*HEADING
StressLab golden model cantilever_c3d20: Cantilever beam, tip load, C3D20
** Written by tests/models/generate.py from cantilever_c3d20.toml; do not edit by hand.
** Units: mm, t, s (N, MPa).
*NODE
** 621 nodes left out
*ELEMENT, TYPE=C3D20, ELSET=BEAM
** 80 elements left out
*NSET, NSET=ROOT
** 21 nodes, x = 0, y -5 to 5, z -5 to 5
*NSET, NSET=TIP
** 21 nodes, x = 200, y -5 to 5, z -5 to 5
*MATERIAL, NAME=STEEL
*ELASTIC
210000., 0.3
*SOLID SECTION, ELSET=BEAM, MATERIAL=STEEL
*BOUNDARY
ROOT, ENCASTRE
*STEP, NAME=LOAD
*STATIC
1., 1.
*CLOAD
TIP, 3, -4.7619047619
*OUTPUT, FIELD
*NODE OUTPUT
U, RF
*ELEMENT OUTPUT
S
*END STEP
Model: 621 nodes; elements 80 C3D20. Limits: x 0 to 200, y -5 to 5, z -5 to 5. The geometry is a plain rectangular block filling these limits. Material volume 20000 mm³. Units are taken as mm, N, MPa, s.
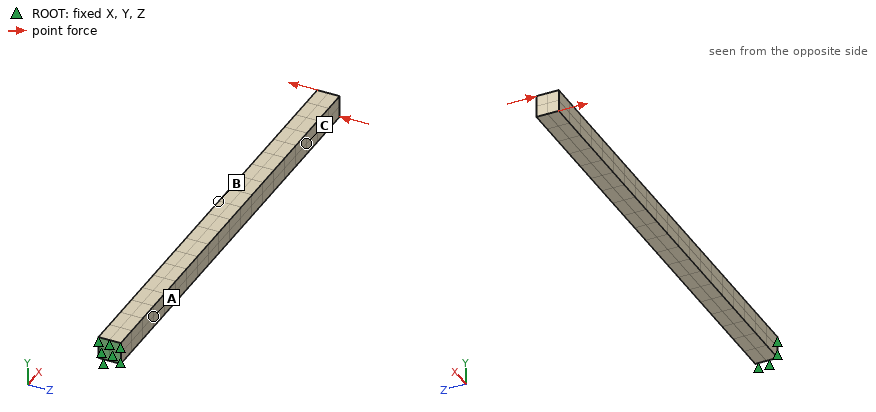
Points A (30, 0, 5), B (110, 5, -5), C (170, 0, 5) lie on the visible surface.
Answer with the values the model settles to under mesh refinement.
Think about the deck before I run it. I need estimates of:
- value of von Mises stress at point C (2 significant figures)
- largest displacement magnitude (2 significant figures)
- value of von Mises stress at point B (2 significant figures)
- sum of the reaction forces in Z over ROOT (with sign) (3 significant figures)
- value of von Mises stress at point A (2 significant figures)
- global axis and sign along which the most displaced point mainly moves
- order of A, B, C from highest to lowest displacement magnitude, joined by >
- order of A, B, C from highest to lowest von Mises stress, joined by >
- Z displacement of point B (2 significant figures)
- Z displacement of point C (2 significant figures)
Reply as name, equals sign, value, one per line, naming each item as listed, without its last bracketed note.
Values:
value of von Mises stress at point C = 18 MPa
largest displacement magnitude = 1.5 mm
value of von Mises stress at point B = 54 MPa
sum of the reaction forces in Z over ROOT (with sign) = 100 N
value of von Mises stress at point A = 100 MPa
global axis and sign along which the most displaced point mainly moves = -Z
order of A, B, C from highest to lowest displacement magnitude, joined by > = C > B > A
order of A, B, C from highest to lowest von Mises stress, joined by > = A > B > C
Z displacement of point B = -0.56 mm
Z displacement of point C = -1.2 mm
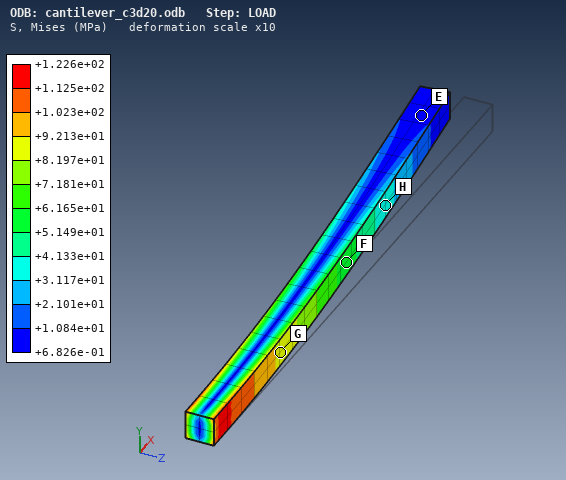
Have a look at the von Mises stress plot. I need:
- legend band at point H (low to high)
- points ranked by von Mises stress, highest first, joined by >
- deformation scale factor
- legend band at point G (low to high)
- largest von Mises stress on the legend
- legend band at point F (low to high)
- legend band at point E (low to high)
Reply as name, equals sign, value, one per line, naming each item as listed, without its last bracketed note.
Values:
legend band at point H = +3.117e+01 to +4.133e+01 MPa
points ranked by von Mises stress, highest first, joined by > = G > F > H > E
deformation scale factor = 10
legend band at point G = +8.197e+01 to +9.213e+01 MPa
largest von Mises stress on the legend = +1.226e+02 MPa
legend band at point F = +5.149e+01 to +6.165e+01 MPa
legend band at point E = +6.826e-01 to +1.084e+01 MPa
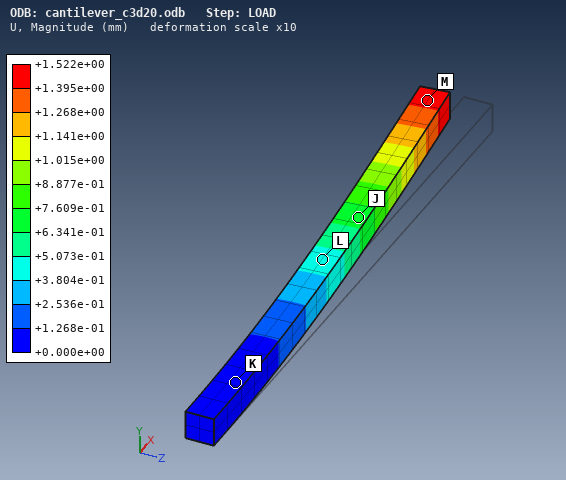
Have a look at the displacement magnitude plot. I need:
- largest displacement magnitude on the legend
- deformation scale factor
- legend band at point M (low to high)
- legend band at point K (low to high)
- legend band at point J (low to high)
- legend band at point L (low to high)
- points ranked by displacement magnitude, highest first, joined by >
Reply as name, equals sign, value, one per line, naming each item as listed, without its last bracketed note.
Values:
largest displacement magnitude on the legend = +1.522e+00 mm
deformation scale factor = 10
legend band at point M = +1.395e+00 to +1.522e+00 mm
legend band at point K = +0.000e+00 to +1.268e-01 mm
legend band at point J = +6.341e-01 to +7.609e-01 mm
legend band at point L = +3.804e-01 to +5.073e-01 mm
points ranked by displacement magnitude, highest first, joined by > = M > J > L > K
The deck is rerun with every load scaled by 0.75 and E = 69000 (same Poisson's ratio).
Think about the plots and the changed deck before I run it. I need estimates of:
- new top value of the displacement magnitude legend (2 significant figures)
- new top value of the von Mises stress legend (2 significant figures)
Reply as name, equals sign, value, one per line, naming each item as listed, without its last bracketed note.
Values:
new top value of the displacement magnitude legend = 3.5 mm
new top value of the von Mises stress legend = 92 MPa
